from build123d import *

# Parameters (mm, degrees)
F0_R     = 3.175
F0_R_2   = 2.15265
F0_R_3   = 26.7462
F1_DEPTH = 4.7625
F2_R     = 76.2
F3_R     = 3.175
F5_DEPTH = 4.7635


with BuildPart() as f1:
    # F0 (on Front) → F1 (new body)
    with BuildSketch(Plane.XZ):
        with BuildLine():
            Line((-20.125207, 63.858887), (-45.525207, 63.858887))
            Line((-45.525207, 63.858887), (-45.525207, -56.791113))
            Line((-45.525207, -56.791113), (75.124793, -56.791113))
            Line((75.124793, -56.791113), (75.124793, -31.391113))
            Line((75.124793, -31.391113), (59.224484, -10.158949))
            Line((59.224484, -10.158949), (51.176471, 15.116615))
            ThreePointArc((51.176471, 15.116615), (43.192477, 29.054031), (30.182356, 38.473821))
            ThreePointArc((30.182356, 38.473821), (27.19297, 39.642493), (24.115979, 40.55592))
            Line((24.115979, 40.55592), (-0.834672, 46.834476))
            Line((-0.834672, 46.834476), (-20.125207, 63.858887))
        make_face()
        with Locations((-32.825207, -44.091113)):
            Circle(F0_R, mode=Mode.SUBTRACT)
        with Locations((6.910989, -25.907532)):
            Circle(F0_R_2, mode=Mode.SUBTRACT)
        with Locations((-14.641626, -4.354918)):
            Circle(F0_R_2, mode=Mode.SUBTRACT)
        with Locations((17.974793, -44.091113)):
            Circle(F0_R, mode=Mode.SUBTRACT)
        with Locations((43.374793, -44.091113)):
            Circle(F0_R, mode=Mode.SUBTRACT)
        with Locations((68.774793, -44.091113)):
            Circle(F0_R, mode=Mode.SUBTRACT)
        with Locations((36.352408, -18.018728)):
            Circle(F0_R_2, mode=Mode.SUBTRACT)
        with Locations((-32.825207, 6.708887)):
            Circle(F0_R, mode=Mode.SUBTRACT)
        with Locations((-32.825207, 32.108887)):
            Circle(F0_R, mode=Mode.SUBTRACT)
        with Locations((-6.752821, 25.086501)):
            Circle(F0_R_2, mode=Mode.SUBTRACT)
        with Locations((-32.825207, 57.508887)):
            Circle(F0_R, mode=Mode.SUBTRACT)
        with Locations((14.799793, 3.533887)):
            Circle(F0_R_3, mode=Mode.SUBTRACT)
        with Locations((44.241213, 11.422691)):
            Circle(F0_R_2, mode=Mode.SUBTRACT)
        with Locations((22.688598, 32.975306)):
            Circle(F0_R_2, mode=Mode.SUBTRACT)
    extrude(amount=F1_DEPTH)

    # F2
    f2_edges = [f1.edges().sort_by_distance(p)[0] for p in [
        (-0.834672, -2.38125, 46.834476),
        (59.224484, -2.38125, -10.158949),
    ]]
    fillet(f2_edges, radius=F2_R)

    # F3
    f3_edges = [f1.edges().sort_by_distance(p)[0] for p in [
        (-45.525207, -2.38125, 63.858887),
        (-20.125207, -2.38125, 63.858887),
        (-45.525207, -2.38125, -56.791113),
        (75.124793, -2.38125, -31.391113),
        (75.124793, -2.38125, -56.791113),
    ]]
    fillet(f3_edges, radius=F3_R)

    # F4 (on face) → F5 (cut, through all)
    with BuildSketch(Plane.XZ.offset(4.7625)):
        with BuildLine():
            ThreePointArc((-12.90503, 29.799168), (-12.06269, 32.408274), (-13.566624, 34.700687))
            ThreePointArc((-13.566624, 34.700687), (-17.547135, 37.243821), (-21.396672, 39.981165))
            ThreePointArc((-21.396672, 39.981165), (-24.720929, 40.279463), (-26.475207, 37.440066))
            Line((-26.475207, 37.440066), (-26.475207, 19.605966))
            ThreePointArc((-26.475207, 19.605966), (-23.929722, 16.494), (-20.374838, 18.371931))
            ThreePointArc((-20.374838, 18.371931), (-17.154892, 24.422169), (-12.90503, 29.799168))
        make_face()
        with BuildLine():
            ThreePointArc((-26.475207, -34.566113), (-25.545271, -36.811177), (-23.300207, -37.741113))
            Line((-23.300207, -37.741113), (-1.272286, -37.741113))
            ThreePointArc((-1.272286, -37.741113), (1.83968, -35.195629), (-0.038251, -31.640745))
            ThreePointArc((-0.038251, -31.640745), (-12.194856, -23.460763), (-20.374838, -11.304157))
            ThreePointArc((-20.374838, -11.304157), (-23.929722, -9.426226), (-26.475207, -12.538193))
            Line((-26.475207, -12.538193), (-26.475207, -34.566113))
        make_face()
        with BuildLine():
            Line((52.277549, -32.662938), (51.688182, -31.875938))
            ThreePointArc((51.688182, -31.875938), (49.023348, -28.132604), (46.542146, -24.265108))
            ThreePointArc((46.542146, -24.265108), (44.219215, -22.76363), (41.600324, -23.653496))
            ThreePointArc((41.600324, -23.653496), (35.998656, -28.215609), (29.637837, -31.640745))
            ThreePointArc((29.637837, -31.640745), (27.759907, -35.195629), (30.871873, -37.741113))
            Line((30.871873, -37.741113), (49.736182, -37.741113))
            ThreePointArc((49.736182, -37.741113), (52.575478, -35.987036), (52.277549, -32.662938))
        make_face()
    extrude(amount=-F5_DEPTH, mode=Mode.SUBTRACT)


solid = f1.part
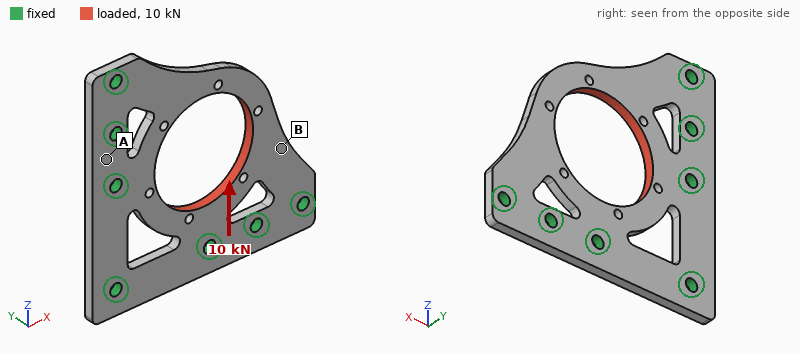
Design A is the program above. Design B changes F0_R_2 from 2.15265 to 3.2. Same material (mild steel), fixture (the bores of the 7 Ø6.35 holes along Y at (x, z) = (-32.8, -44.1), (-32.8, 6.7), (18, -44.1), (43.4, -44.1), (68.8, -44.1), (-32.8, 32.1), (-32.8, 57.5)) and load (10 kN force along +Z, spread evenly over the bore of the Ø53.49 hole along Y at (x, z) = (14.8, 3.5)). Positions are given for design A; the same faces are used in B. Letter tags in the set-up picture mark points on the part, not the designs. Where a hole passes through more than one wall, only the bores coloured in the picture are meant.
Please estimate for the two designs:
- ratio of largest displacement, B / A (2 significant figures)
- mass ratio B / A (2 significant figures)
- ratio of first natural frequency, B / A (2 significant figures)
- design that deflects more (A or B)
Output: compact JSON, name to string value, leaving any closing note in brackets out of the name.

{"ratio of largest displacement, B / A": "1.3", "mass ratio B / A": "0.99", "ratio of first natural frequency, B / A": "1.00", "design that deflects more": "B"}
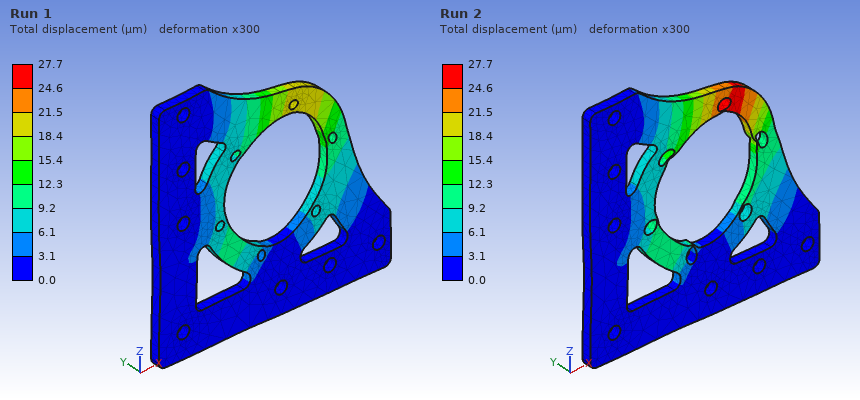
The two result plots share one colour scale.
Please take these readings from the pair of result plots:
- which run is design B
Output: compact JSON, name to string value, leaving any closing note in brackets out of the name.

{"which run is design B": "Run 2"}
